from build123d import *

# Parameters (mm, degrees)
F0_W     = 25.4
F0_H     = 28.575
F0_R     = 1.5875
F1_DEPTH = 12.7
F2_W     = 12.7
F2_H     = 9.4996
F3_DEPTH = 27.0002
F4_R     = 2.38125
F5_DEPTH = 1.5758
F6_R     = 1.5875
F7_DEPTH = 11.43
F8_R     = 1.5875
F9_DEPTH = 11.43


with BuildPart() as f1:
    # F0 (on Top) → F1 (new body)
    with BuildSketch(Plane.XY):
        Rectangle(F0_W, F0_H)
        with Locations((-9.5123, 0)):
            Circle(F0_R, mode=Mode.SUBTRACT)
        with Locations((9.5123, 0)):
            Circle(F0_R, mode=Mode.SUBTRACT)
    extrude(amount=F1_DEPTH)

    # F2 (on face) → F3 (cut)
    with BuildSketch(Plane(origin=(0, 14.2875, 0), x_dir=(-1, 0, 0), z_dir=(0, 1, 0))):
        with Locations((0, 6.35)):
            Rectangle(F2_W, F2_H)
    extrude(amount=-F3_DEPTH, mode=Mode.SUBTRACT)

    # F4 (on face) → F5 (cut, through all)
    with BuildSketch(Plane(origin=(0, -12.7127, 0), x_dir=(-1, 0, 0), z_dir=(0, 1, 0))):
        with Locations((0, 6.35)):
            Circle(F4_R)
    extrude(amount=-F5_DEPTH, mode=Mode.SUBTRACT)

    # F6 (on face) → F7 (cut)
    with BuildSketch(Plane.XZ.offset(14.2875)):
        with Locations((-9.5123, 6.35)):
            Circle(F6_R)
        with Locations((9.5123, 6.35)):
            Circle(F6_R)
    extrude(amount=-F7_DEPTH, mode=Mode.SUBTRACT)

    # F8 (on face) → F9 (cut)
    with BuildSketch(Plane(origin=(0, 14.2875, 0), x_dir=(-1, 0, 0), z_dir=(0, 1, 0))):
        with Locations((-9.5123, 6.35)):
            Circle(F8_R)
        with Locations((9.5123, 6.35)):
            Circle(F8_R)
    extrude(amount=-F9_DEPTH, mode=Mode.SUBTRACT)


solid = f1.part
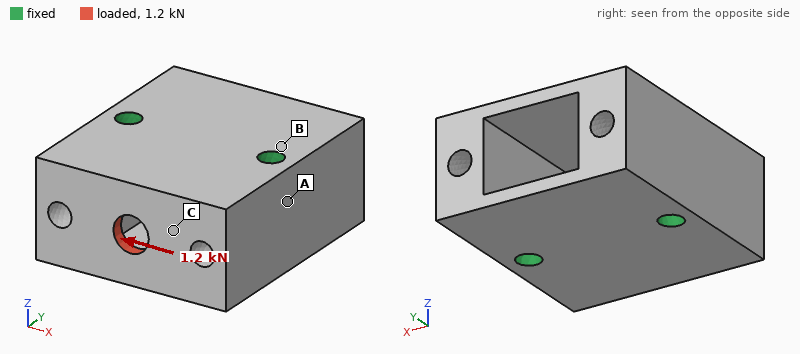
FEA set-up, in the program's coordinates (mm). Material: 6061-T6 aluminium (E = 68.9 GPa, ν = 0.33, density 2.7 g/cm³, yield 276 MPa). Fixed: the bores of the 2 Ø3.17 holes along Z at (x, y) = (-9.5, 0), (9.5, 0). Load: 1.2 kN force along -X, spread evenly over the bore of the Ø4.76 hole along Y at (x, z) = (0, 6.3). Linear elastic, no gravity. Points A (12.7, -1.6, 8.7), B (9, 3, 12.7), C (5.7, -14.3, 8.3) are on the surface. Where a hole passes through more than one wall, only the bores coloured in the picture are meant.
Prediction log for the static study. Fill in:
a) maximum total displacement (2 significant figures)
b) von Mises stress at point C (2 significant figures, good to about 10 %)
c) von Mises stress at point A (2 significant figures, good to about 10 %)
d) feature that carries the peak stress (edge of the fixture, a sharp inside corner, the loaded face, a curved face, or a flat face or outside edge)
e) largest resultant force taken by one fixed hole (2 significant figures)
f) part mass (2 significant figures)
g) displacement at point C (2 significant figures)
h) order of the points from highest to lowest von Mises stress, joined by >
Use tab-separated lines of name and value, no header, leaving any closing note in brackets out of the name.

maximum total displacement	11 µm
von Mises stress at point C	33 MPa
von Mises stress at point A	19 MPa
feature that carries the peak stress	the loaded face
largest resultant force taken by one fixed hole	890 N
part mass	14 g
displacement at point C	9.1 µm
order of the points from highest to lowest von Mises stress, joined by >	C > A > B
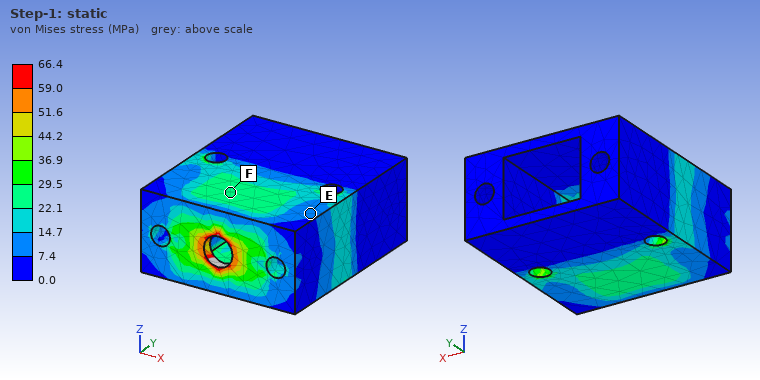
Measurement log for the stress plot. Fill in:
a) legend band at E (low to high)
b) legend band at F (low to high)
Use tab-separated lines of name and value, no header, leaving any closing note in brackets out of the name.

legend band at E	7.4 to 14.7 MPa
legend band at F	22.1 to 29.5 MPa
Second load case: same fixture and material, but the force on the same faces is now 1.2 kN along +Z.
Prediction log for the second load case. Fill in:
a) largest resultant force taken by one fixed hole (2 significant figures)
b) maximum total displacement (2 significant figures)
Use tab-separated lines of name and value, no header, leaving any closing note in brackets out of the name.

largest resultant force taken by one fixed hole	600 N
maximum total displacement	23 µm
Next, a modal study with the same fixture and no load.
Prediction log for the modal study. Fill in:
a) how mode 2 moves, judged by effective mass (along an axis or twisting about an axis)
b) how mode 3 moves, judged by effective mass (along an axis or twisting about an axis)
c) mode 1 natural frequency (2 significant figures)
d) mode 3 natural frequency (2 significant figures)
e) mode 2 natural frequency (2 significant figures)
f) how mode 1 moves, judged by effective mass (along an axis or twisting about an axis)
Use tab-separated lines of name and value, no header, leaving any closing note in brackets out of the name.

how mode 2 moves, judged by effective mass	along Z
how mode 3 moves, judged by effective mass	along X
mode 1 natural frequency	29 kHz
mode 3 natural frequency	36 kHz
mode 2 natural frequency	31 kHz
how mode 1 moves, judged by effective mass	twisting about X
